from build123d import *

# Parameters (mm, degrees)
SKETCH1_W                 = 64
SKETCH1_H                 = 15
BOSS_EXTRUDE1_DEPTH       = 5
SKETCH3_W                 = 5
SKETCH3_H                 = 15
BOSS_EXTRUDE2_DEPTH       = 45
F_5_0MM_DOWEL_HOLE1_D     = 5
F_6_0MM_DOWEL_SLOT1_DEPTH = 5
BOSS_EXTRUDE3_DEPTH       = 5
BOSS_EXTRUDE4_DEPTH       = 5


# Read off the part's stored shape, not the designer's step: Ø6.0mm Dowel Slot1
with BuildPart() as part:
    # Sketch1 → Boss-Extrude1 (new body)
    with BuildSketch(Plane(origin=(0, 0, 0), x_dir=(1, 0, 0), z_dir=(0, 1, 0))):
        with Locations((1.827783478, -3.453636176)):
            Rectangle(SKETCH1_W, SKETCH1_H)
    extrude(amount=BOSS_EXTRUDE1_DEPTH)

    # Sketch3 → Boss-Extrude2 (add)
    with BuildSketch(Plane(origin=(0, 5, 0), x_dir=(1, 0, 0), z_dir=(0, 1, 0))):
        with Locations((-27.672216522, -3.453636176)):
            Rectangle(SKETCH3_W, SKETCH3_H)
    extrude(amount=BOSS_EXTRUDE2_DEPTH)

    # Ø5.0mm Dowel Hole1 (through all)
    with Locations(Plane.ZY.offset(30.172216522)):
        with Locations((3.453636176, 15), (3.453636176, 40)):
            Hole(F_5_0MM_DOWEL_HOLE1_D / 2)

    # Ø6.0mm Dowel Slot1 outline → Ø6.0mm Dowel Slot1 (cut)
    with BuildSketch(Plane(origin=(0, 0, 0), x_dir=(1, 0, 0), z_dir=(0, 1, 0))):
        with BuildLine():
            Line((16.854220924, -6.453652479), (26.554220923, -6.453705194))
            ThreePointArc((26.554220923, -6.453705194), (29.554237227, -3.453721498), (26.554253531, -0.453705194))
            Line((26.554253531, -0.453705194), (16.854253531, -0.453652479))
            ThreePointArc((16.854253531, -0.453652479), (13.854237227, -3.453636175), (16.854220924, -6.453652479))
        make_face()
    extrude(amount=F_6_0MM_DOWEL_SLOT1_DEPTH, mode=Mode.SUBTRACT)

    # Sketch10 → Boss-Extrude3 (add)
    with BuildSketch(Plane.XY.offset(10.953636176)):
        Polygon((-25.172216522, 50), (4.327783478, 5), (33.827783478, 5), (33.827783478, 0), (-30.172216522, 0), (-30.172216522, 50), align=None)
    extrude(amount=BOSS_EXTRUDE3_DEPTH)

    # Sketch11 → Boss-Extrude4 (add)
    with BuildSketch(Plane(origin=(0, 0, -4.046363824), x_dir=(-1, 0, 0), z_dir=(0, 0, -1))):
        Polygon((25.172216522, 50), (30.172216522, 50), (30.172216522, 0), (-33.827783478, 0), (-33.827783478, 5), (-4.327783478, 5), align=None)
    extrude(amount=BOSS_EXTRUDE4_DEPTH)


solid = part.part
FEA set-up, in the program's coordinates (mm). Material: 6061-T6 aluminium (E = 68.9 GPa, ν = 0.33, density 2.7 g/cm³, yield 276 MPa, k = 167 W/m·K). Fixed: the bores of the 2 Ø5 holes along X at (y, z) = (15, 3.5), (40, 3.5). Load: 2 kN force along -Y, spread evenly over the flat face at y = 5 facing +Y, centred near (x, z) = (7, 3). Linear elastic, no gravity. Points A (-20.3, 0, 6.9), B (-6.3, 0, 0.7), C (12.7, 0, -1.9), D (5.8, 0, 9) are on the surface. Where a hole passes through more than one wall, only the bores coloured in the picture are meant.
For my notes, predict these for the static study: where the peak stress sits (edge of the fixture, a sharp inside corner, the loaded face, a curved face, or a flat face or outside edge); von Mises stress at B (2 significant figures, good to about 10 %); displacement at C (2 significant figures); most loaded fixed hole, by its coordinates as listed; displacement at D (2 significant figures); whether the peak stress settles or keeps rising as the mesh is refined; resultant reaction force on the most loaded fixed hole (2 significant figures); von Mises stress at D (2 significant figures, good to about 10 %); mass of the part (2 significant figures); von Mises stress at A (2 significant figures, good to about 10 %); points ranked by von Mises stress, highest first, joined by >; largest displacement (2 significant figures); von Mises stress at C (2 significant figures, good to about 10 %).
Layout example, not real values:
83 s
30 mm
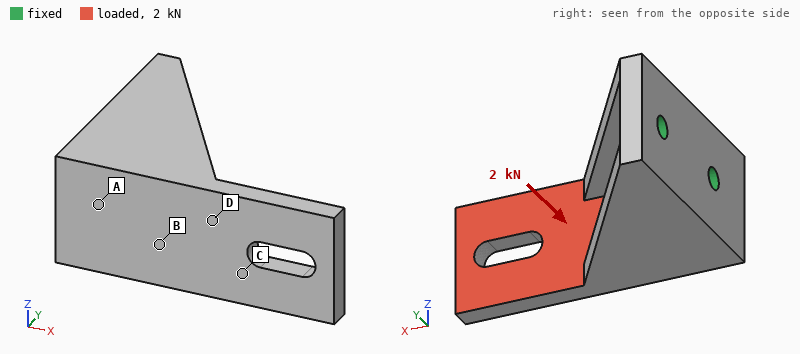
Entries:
edge of the fixture
58 MPa
0.21 mm
(40, 3.5)
0.13 mm
keeps rising
2.8 kN
140 MPa
53 g
20 MPa
D > C > B > A
0.58 mm
110 MPa
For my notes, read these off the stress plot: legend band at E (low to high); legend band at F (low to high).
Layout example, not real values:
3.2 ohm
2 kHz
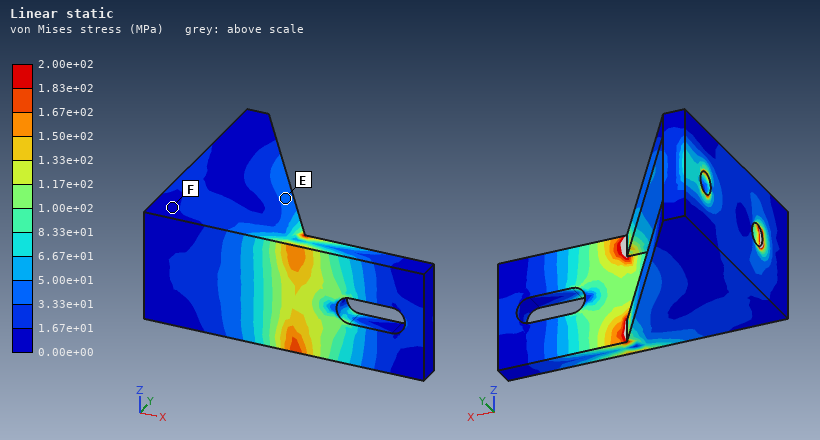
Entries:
3.33e+01 to 5.00e+01 MPa
0.00e+00 to 1.67e+01 MPa
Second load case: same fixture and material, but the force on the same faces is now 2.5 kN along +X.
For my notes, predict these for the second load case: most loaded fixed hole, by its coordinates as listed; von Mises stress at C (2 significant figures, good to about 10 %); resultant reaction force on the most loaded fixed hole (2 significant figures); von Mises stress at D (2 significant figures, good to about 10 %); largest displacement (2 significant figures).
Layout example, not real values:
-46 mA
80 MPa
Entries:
(15, 3.5)
20 MPa
3.1 kN
21 MPa
53 µm
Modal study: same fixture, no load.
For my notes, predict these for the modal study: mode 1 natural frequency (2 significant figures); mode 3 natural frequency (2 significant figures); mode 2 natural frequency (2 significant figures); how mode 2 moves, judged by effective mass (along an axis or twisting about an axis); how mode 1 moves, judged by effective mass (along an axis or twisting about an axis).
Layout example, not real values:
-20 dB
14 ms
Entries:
2300 Hz
7500 Hz
3000 Hz
along Y
along Z
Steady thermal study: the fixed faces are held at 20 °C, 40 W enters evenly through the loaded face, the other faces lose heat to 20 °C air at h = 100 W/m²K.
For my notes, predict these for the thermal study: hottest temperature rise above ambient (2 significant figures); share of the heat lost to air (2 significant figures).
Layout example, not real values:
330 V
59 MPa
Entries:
42 K
26 %
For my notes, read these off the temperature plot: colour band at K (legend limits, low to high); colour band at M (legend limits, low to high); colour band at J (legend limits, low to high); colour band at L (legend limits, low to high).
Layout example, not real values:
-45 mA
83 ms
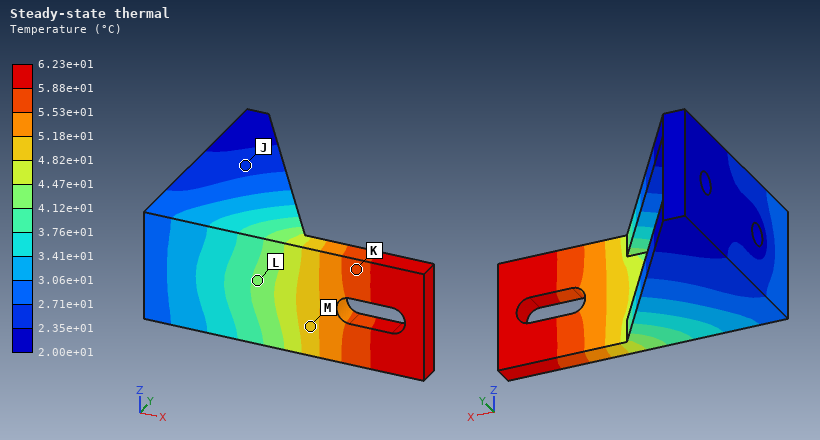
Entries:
5.53e+01 to 5.88e+01 °C
4.82e+01 to 5.18e+01 °C
2.35e+01 to 2.71e+01 °C
4.12e+01 to 4.47e+01 °C
